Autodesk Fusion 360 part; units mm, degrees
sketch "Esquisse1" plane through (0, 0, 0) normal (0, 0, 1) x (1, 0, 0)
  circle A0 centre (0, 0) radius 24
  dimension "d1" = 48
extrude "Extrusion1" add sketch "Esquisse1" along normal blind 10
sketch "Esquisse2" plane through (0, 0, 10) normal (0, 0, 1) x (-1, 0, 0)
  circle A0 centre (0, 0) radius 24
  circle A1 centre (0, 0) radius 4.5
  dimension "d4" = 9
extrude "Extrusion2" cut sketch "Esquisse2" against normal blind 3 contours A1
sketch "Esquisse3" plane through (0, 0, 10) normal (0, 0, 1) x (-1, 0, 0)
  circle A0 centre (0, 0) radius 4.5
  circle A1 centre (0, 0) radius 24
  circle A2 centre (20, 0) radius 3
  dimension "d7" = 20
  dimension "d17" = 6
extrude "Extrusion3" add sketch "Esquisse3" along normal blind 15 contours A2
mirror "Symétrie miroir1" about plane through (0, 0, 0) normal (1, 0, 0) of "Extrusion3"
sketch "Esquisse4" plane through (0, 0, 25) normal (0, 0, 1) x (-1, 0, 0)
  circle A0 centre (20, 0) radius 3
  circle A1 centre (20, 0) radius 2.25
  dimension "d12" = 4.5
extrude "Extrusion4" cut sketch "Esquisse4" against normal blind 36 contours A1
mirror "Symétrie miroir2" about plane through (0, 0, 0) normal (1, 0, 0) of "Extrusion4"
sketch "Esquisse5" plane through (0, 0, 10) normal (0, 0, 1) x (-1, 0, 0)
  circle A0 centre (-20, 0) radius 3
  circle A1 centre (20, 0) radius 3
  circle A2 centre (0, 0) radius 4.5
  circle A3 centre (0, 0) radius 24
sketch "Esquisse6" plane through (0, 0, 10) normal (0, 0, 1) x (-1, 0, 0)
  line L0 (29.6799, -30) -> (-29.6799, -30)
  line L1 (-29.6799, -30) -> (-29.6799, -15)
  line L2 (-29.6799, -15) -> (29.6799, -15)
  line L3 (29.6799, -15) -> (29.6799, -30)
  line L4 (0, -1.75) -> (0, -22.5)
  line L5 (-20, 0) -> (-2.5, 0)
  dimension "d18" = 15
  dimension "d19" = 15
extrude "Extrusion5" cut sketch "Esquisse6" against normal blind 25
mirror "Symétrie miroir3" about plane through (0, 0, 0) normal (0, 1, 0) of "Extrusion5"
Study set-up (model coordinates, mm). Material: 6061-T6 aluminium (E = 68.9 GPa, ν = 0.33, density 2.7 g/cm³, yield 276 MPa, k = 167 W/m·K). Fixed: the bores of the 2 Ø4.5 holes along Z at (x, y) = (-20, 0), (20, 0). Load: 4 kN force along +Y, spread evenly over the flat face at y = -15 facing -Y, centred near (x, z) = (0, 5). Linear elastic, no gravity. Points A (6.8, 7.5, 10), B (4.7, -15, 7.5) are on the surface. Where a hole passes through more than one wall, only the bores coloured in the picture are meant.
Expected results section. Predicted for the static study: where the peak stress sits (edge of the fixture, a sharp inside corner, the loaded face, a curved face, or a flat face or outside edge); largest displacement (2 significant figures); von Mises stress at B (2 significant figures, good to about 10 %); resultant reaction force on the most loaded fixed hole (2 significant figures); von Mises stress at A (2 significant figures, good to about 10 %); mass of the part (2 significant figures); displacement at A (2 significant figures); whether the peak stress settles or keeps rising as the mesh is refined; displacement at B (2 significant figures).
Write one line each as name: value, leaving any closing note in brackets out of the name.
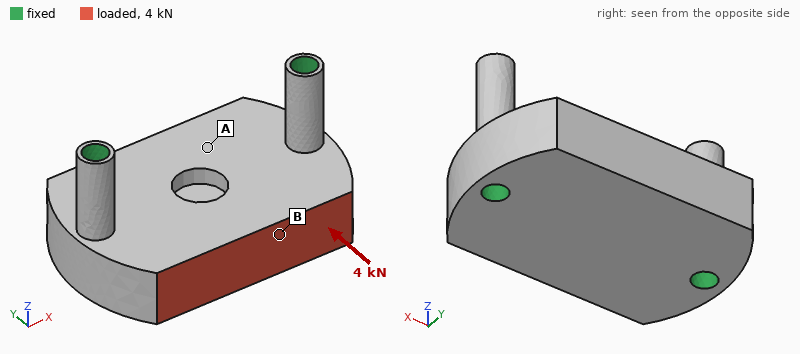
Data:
where the peak stress sits: edge of the fixture
largest displacement: 6.5 µm
von Mises stress at B: 14 MPa
resultant reaction force on the most loaded fixed hole: 2.0 kN
von Mises stress at A: 6.6 MPa
mass of the part: 36 g
displacement at A: 3.7 µm
whether the peak stress settles or keeps rising as the mesh is refined: keeps rising
displacement at B: 6.0 µm
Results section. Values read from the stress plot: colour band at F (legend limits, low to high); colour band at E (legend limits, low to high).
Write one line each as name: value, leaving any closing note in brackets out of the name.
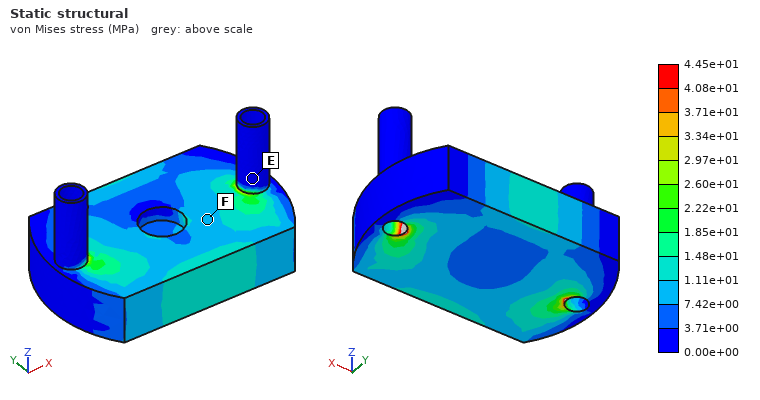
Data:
colour band at F: 7.42e+00 to 1.11e+01 MPa
colour band at E: 0.00e+00 to 3.71e+00 MPa
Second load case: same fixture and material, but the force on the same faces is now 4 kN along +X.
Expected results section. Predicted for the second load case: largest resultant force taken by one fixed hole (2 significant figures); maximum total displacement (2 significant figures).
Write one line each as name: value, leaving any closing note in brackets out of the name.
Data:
largest resultant force taken by one fixed hole: 2.4 kN
maximum total displacement: 7.5 µm
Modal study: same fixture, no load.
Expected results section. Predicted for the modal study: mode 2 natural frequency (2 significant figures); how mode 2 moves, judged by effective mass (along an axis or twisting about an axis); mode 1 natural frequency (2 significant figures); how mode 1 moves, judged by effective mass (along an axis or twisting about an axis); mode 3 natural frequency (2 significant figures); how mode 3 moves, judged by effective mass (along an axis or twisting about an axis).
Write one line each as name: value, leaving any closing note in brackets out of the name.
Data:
mode 2 natural frequency: 19 kHz
how mode 2 moves, judged by effective mass: along Z
mode 1 natural frequency: 18 kHz
how mode 1 moves, judged by effective mass: twisting about X
mode 3 natural frequency: 28 kHz
how mode 3 moves, judged by effective mass: along Y
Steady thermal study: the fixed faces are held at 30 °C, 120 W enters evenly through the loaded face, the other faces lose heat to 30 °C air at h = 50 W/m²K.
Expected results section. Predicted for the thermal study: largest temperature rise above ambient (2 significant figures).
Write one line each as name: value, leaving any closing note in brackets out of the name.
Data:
largest temperature rise above ambient: 38 K
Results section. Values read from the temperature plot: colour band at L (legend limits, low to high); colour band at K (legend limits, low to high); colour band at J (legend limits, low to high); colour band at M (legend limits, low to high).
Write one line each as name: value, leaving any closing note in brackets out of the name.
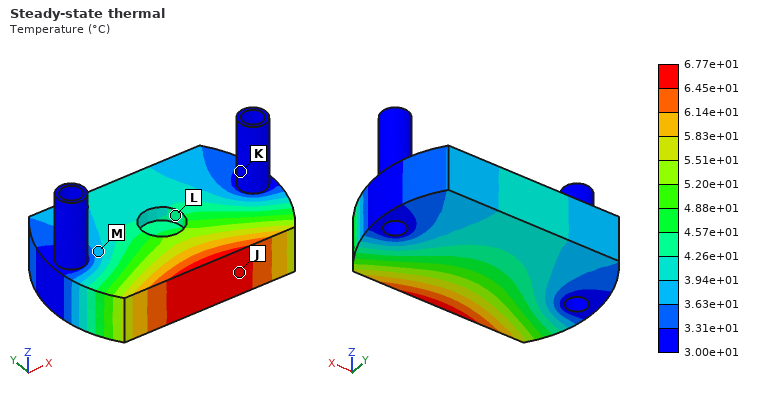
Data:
colour band at L: 4.26e+01 to 4.57e+01 °C
colour band at K: 3.00e+01 to 3.31e+01 °C
colour band at J: 6.45e+01 to 6.77e+01 °C
colour band at M: 3.63e+01 to 3.94e+01 °C
